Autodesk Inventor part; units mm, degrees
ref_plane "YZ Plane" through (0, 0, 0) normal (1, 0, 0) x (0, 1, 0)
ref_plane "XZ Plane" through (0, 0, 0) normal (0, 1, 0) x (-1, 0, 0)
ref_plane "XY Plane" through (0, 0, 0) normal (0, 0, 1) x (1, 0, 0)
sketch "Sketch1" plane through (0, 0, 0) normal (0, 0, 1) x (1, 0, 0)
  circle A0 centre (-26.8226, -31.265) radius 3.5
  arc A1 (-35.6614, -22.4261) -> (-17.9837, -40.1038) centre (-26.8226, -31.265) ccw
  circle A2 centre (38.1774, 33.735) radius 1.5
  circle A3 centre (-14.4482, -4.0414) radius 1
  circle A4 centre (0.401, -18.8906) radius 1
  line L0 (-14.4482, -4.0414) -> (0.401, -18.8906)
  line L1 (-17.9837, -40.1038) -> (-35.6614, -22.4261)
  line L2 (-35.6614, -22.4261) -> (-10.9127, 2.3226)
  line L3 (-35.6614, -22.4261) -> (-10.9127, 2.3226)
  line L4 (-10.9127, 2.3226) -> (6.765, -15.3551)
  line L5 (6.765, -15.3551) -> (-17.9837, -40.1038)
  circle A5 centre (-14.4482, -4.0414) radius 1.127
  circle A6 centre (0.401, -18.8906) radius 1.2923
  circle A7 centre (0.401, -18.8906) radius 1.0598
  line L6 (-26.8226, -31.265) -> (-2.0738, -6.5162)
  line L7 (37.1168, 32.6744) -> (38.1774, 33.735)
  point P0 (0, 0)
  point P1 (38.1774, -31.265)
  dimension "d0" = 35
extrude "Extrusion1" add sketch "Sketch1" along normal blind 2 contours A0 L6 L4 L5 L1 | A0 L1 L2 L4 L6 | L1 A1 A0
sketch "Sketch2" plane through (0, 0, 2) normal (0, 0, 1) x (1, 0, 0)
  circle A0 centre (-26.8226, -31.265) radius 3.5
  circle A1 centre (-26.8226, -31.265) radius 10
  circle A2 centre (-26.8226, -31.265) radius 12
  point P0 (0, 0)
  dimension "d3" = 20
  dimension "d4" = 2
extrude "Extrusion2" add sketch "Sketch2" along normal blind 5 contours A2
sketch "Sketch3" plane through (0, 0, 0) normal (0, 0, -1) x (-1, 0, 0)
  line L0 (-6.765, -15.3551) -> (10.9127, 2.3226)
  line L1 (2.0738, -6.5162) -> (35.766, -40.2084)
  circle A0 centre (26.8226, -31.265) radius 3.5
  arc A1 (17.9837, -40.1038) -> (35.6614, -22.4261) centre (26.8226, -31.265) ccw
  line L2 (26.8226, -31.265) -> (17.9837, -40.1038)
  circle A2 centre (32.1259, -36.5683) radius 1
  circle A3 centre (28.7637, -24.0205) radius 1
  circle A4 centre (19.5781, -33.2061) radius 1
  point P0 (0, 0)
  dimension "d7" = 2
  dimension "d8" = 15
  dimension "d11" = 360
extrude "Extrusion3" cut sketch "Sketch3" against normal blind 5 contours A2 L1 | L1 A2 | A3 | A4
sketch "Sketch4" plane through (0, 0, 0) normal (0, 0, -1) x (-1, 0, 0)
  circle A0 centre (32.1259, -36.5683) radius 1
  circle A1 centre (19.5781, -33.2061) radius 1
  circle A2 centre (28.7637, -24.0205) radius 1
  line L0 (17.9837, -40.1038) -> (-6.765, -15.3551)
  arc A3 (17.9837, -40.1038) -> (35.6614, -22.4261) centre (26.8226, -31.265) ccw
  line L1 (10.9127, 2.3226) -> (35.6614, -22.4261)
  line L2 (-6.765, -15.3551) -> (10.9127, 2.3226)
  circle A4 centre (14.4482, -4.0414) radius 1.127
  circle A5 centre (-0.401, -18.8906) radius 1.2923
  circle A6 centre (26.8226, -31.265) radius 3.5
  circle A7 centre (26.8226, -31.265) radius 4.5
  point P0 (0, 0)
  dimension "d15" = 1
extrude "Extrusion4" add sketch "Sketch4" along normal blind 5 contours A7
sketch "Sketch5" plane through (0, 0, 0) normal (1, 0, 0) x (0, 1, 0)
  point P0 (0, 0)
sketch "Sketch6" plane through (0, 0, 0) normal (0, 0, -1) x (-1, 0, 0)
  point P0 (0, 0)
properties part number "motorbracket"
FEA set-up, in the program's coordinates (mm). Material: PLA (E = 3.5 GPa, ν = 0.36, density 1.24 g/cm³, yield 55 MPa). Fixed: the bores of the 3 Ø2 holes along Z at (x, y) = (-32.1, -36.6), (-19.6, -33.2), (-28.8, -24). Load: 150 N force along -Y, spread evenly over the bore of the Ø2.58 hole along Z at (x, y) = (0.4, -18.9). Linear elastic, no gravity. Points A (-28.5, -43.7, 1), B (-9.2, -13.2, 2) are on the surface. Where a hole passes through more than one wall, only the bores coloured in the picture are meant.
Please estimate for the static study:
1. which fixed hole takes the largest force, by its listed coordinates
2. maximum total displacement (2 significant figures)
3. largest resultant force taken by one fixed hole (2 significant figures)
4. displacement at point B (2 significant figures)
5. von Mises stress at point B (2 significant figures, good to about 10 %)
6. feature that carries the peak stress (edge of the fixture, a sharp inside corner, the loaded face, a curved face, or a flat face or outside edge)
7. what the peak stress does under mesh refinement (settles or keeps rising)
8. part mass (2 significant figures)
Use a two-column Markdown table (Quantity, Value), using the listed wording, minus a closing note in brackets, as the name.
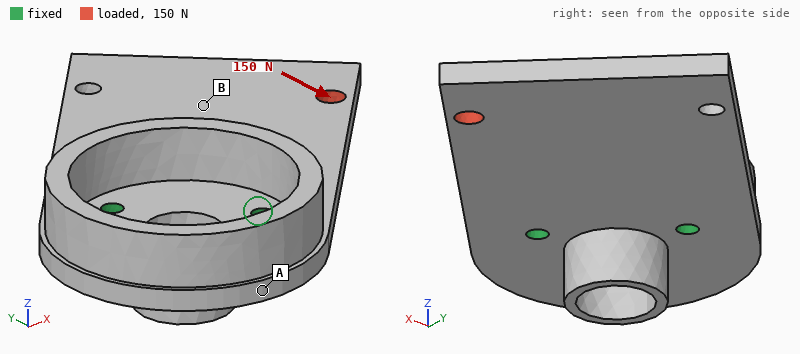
| Quantity | Value |
|---|---|
| which fixed hole takes the largest force, by its listed coordinates | (-19.6, -33.2) |
| maximum total displacement | 0.27 mm |
| largest resultant force taken by one fixed hole | 280 N |
| displacement at point B | 0.15 mm |
| von Mises stress at point B | 5.3 MPa |
| feature that carries the peak stress | edge of the fixture |
| what the peak stress does under mesh refinement | keeps rising |
| part mass | 3.6 g |
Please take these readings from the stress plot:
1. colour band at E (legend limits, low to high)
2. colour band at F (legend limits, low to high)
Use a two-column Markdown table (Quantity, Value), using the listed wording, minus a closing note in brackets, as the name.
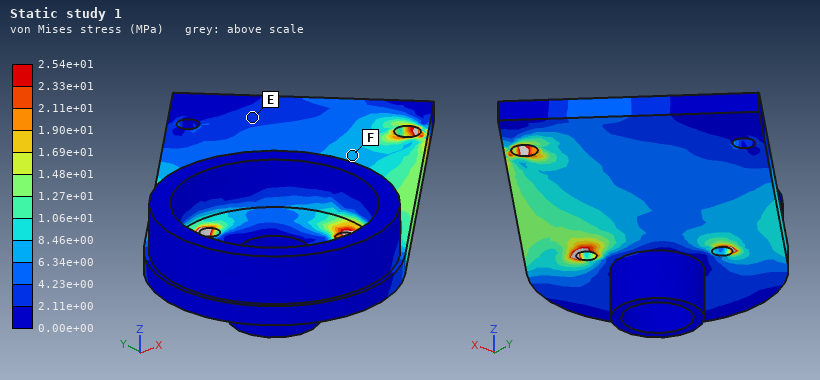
| Quantity | Value |
|---|---|
| colour band at E | 2.11e+00 to 4.23e+00 MPa |
| colour band at F | 6.34e+00 to 8.46e+00 MPa |
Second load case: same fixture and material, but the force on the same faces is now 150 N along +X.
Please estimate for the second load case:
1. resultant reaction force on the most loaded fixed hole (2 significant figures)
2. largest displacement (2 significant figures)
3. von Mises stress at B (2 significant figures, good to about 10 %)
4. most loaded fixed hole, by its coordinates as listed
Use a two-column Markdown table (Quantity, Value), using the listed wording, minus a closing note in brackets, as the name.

| Quantity | Value |
|---|---|
| resultant reaction force on the most loaded fixed hole | 150 N |
| largest displacement | 0.11 mm |
| von Mises stress at B | 3.8 MPa |
| most loaded fixed hole, by its coordinates as listed | (-28.8, -24) |
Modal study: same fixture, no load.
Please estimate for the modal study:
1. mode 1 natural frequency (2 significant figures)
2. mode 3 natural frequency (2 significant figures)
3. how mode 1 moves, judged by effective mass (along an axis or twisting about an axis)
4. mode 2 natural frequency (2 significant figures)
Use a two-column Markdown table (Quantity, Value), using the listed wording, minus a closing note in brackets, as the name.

| Quantity | Value |
|---|---|
| mode 1 natural frequency | 720 Hz |
| mode 3 natural frequency | 3700 Hz |
| how mode 1 moves, judged by effective mass | along Z |
| mode 2 natural frequency | 1700 Hz |
